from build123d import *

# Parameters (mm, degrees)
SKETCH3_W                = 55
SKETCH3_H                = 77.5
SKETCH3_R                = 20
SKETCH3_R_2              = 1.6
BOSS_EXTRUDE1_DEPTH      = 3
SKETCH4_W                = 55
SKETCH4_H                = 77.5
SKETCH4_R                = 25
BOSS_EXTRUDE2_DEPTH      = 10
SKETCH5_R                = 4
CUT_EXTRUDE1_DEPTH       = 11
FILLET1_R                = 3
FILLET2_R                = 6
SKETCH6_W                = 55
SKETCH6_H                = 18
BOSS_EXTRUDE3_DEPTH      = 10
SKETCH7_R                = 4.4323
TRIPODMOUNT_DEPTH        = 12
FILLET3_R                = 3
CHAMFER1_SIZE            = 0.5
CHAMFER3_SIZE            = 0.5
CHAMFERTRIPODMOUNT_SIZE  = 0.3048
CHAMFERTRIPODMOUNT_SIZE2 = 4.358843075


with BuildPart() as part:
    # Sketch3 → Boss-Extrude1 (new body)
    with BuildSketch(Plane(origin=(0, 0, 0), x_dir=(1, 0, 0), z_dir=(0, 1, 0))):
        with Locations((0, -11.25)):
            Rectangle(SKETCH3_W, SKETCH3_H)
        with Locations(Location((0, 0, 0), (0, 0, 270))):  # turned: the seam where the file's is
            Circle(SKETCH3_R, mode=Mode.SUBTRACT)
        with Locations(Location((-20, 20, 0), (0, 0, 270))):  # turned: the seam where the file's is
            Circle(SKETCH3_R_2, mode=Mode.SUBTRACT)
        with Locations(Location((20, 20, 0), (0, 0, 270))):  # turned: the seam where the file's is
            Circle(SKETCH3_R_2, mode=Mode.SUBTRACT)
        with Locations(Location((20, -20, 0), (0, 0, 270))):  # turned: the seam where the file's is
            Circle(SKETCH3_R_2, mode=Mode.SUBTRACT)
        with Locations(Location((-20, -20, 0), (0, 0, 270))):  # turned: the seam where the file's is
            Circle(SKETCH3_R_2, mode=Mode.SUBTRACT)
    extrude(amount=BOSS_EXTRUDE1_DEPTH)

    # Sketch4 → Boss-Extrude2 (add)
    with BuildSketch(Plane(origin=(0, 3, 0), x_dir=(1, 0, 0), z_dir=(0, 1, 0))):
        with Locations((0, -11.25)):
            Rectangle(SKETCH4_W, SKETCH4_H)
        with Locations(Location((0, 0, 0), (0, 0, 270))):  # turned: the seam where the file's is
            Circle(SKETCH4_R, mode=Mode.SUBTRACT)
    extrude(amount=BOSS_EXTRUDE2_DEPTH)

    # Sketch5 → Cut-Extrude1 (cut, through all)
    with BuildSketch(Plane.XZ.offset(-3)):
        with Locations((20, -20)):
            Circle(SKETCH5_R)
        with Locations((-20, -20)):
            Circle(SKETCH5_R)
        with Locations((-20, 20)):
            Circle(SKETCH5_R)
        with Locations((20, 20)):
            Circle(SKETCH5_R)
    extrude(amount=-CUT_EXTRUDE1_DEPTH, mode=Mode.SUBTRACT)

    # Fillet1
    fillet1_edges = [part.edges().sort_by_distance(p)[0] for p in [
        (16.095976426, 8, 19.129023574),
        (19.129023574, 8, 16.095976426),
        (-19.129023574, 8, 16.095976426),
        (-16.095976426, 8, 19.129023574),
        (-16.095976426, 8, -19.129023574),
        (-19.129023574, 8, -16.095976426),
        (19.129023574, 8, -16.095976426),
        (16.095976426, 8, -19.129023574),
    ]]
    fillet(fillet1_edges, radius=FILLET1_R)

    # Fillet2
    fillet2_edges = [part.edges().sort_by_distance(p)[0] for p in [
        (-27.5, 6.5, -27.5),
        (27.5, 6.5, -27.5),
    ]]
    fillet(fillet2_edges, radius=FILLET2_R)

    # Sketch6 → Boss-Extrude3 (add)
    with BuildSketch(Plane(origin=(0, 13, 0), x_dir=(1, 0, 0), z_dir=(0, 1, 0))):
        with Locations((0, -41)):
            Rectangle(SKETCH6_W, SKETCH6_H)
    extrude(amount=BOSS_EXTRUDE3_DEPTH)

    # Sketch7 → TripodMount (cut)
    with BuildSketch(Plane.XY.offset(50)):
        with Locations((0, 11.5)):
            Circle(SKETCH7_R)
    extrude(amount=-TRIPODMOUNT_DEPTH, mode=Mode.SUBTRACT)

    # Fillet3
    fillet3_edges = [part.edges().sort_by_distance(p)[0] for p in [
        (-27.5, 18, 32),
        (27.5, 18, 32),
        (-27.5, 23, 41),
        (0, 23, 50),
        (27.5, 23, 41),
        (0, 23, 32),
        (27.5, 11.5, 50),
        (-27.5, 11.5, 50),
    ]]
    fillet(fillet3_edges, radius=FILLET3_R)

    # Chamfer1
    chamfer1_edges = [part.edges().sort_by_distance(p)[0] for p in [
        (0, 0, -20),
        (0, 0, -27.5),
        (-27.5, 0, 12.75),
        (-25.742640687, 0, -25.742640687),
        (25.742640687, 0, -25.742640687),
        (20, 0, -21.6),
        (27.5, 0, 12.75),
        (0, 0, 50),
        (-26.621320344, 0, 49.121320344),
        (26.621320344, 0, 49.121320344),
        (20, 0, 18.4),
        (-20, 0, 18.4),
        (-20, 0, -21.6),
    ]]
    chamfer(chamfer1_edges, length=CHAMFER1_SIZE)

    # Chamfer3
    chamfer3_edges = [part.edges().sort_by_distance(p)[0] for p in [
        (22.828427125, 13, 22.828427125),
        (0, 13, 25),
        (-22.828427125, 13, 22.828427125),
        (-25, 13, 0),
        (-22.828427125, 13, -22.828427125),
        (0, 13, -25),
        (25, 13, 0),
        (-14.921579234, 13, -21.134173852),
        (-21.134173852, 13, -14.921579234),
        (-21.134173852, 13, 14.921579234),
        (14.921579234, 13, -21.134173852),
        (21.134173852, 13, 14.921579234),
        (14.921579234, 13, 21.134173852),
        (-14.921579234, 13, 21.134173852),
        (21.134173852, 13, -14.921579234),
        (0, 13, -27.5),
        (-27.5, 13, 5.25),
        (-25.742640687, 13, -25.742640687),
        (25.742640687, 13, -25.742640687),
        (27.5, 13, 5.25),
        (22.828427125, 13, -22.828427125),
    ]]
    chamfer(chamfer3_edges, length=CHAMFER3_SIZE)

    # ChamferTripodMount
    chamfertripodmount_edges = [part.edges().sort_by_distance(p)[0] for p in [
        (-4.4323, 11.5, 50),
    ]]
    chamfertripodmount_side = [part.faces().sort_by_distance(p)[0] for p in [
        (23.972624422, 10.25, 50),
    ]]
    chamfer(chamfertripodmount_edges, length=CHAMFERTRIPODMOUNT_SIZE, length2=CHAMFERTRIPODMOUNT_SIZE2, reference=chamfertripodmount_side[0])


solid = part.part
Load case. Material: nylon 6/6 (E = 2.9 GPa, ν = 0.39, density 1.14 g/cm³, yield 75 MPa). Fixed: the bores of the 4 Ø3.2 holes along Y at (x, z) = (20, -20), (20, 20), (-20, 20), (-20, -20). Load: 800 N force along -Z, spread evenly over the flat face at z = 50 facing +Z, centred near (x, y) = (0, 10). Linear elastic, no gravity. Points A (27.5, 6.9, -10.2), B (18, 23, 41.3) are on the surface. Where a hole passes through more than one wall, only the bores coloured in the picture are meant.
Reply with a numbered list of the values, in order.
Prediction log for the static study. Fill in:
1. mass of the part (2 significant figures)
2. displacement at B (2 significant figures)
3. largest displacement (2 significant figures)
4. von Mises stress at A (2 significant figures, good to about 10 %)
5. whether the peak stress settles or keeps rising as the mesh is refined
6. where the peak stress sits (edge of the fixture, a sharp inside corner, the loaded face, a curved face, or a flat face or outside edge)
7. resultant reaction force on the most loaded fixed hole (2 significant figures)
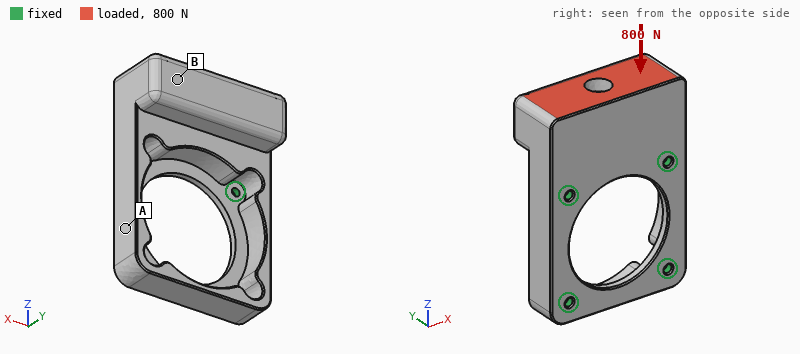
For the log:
1. 44 g
2. 0.56 mm
3. 0.67 mm
4. 5.4 MPa
5. keeps rising
6. edge of the fixture
7. 280 N
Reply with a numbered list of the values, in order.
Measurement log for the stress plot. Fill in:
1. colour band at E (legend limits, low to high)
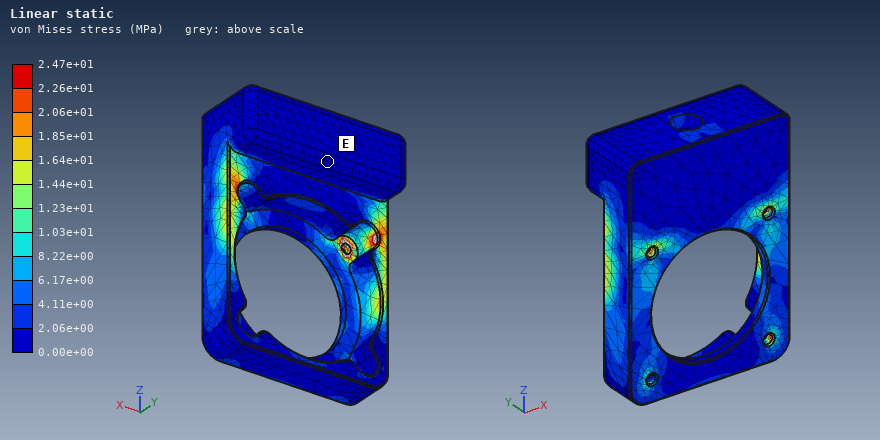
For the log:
1. 0.00e+00 to 2.06e+00 MPa
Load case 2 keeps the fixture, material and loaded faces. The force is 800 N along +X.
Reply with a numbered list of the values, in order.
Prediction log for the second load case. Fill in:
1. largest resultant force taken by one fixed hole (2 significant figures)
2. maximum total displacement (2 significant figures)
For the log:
1. 640 N
2. 0.15 mm
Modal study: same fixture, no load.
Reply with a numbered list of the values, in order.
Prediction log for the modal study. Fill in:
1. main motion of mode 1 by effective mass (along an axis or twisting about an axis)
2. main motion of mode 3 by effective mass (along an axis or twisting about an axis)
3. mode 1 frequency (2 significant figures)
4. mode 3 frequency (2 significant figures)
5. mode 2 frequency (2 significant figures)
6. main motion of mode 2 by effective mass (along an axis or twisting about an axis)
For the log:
1. along Y
2. along X
3. 760 Hz
4. 3000 Hz
5. 2100 Hz
6. along X
